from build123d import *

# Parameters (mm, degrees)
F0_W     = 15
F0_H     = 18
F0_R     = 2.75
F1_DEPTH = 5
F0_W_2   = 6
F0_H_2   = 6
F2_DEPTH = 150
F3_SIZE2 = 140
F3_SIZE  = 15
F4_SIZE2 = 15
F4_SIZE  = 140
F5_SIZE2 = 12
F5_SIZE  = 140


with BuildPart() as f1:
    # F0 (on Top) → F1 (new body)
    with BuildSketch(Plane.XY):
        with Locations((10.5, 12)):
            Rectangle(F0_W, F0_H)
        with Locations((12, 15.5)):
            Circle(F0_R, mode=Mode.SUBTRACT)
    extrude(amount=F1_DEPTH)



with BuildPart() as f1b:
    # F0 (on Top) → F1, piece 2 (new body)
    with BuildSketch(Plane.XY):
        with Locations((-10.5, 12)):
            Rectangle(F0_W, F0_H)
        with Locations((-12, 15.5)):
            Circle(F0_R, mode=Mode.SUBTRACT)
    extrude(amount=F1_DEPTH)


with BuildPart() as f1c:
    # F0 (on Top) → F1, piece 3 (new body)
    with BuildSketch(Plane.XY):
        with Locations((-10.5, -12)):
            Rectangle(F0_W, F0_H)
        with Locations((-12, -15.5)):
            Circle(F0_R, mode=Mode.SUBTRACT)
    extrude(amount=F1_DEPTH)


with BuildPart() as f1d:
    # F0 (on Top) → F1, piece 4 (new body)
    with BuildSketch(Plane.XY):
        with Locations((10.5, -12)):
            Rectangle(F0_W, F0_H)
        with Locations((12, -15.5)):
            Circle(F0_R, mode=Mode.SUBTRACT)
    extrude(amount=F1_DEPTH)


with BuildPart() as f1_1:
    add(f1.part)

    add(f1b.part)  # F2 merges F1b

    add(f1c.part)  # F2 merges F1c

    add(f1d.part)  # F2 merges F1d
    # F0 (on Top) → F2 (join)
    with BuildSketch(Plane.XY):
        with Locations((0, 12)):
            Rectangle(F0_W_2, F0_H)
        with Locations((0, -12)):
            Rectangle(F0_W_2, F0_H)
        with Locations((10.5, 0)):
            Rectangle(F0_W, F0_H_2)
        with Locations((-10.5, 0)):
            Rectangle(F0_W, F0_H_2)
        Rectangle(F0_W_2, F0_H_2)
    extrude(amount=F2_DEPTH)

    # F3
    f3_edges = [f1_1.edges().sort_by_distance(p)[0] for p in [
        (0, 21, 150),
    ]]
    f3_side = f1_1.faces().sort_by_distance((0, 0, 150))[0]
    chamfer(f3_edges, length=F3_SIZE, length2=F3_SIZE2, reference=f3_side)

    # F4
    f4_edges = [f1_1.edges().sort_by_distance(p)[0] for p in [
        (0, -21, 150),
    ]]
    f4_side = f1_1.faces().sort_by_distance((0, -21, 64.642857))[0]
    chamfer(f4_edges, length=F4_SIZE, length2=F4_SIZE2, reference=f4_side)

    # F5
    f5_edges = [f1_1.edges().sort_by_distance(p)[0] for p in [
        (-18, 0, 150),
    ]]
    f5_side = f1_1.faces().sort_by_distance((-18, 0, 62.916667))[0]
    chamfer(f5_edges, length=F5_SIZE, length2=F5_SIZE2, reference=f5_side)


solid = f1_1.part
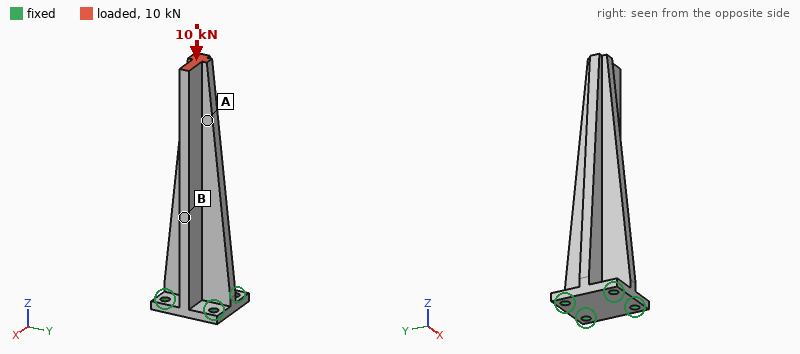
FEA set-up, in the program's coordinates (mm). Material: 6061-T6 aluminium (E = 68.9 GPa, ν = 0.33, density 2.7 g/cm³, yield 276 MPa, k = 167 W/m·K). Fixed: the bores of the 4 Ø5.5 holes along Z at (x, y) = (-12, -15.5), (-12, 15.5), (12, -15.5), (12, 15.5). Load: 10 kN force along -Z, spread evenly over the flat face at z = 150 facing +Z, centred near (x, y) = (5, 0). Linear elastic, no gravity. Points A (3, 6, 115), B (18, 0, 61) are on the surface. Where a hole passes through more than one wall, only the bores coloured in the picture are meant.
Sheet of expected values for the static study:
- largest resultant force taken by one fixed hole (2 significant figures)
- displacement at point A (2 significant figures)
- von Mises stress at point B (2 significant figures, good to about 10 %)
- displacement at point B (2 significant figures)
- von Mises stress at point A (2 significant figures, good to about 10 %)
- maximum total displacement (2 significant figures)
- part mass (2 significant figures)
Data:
3.5 kN
0.36 mm
65 MPa
0.17 mm
41 MPa
0.56 mm
140 g
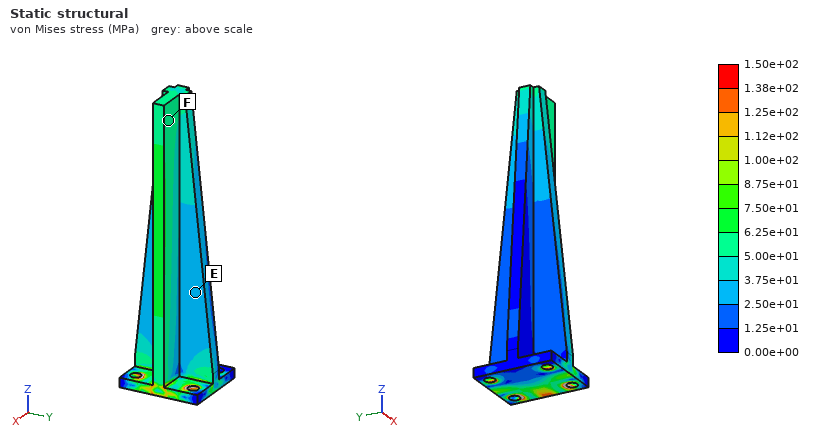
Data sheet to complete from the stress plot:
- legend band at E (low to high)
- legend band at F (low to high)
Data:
2.50e+01 to 3.75e+01 MPa
5.00e+01 to 6.25e+01 MPa
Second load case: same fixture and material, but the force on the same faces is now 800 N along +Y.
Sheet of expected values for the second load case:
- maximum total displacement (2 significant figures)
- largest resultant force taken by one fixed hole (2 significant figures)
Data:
0.99 mm
2.0 kN
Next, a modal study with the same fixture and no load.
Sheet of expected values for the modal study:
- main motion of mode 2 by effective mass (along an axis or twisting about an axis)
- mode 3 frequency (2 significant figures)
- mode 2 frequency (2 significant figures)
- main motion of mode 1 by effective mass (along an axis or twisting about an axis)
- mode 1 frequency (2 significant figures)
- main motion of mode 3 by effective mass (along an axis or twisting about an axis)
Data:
along Y
2800 Hz
1000 Hz
along X
810 Hz
twisting about Z
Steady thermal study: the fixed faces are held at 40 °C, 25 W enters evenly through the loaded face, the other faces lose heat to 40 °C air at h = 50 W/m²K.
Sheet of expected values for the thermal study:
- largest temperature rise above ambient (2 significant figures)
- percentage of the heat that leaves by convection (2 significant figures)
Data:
53 K
57 %
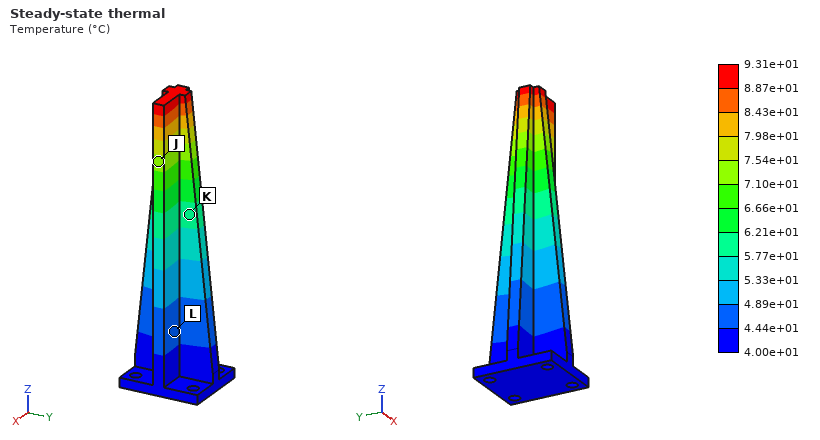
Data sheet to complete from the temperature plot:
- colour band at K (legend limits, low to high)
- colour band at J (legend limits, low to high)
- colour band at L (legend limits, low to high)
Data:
5.77e+01 to 6.21e+01 °C
7.10e+01 to 7.54e+01 °C
4.44e+01 to 4.89e+01 °C
